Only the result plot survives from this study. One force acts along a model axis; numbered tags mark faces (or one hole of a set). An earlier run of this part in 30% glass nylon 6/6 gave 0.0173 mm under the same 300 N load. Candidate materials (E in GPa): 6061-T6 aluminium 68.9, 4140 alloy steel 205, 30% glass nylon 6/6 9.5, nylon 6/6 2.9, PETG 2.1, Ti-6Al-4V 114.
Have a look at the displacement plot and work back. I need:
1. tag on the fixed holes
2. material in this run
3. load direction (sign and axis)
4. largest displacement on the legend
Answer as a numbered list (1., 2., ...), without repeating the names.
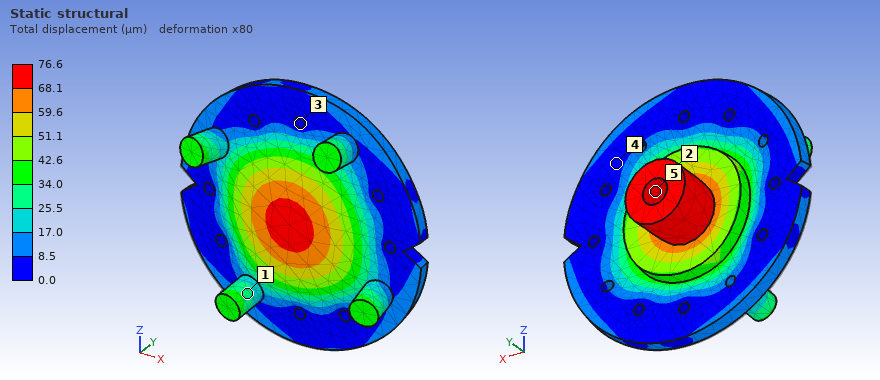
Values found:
1. 3
2. PETG
3. -Y
4. 76.6 µm
